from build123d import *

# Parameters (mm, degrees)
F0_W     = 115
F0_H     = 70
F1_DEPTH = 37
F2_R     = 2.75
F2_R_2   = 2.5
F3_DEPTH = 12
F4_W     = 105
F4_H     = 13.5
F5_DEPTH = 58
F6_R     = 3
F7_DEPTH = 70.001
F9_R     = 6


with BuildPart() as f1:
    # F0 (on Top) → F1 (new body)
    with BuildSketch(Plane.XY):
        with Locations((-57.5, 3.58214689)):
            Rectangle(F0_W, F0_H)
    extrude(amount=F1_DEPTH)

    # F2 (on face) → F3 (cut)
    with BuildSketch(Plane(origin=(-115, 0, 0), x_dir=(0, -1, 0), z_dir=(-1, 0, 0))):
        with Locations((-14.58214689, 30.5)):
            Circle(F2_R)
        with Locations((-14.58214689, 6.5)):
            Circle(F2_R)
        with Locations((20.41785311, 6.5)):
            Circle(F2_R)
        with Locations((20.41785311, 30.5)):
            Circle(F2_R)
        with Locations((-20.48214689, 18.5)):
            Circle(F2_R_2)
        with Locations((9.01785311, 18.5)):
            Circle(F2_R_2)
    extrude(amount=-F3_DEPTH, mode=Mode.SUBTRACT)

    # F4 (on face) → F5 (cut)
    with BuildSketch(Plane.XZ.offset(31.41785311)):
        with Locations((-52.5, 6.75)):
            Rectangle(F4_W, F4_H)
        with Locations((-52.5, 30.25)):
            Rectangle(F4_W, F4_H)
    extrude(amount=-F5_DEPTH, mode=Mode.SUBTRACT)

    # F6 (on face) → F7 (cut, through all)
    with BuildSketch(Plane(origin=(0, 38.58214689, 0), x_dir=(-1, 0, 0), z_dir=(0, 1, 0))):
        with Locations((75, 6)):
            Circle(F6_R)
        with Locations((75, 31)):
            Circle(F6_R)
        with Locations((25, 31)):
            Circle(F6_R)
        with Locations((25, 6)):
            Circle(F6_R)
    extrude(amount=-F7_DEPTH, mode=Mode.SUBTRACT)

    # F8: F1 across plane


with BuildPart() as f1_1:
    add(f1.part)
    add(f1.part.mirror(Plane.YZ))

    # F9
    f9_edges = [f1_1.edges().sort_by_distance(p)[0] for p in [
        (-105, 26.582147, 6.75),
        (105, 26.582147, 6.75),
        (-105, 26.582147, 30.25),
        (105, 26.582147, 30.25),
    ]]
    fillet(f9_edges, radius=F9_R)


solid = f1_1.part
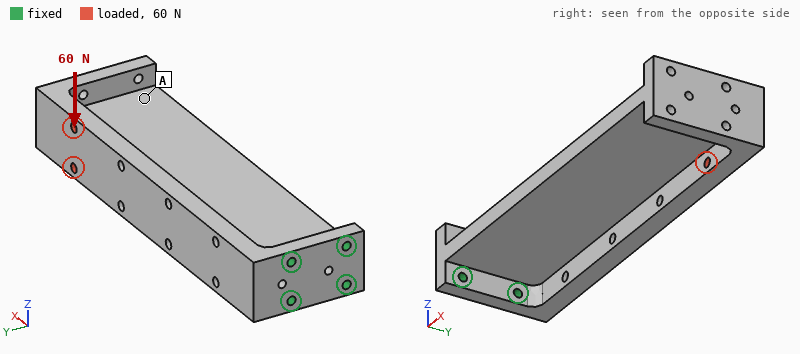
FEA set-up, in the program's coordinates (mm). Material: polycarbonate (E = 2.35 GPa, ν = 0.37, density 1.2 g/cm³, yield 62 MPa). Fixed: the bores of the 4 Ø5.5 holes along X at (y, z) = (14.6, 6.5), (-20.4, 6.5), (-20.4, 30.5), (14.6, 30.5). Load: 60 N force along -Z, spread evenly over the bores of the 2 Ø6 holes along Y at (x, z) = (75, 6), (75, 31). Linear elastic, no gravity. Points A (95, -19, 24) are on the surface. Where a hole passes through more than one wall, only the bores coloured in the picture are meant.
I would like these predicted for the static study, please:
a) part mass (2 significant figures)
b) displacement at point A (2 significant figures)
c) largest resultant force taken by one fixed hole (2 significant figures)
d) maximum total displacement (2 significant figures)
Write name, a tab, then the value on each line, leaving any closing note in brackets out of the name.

part mass	310 g
displacement at point A	1.9 mm
largest resultant force taken by one fixed hole	370 N
maximum total displacement	2.3 mm
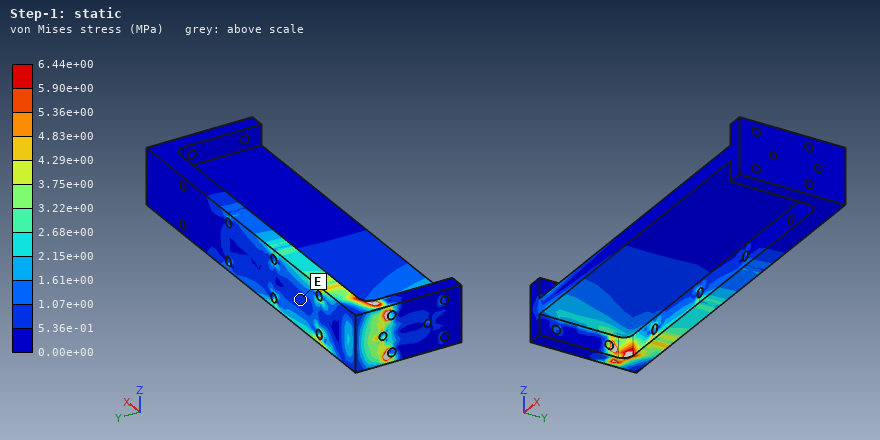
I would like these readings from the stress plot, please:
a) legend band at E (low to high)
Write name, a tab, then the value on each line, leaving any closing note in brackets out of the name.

legend band at E	5.36e-01 to 1.07e+00 MPa
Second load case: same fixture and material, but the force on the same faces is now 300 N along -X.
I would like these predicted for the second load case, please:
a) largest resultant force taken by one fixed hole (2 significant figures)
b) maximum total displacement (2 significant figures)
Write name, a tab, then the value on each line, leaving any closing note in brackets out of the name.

largest resultant force taken by one fixed hole	200 N
maximum total displacement	0.29 mm
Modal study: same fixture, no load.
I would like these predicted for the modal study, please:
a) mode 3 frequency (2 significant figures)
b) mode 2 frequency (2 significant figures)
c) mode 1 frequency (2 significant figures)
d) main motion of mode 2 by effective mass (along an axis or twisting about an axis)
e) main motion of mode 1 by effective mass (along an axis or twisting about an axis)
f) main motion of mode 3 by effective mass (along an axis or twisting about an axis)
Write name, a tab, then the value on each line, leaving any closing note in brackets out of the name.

mode 3 frequency	260 Hz
mode 2 frequency	200 Hz
mode 1 frequency	75 Hz
main motion of mode 2 by effective mass	along Y
main motion of mode 1 by effective mass	along Z
main motion of mode 3 by effective mass	twisting about X
